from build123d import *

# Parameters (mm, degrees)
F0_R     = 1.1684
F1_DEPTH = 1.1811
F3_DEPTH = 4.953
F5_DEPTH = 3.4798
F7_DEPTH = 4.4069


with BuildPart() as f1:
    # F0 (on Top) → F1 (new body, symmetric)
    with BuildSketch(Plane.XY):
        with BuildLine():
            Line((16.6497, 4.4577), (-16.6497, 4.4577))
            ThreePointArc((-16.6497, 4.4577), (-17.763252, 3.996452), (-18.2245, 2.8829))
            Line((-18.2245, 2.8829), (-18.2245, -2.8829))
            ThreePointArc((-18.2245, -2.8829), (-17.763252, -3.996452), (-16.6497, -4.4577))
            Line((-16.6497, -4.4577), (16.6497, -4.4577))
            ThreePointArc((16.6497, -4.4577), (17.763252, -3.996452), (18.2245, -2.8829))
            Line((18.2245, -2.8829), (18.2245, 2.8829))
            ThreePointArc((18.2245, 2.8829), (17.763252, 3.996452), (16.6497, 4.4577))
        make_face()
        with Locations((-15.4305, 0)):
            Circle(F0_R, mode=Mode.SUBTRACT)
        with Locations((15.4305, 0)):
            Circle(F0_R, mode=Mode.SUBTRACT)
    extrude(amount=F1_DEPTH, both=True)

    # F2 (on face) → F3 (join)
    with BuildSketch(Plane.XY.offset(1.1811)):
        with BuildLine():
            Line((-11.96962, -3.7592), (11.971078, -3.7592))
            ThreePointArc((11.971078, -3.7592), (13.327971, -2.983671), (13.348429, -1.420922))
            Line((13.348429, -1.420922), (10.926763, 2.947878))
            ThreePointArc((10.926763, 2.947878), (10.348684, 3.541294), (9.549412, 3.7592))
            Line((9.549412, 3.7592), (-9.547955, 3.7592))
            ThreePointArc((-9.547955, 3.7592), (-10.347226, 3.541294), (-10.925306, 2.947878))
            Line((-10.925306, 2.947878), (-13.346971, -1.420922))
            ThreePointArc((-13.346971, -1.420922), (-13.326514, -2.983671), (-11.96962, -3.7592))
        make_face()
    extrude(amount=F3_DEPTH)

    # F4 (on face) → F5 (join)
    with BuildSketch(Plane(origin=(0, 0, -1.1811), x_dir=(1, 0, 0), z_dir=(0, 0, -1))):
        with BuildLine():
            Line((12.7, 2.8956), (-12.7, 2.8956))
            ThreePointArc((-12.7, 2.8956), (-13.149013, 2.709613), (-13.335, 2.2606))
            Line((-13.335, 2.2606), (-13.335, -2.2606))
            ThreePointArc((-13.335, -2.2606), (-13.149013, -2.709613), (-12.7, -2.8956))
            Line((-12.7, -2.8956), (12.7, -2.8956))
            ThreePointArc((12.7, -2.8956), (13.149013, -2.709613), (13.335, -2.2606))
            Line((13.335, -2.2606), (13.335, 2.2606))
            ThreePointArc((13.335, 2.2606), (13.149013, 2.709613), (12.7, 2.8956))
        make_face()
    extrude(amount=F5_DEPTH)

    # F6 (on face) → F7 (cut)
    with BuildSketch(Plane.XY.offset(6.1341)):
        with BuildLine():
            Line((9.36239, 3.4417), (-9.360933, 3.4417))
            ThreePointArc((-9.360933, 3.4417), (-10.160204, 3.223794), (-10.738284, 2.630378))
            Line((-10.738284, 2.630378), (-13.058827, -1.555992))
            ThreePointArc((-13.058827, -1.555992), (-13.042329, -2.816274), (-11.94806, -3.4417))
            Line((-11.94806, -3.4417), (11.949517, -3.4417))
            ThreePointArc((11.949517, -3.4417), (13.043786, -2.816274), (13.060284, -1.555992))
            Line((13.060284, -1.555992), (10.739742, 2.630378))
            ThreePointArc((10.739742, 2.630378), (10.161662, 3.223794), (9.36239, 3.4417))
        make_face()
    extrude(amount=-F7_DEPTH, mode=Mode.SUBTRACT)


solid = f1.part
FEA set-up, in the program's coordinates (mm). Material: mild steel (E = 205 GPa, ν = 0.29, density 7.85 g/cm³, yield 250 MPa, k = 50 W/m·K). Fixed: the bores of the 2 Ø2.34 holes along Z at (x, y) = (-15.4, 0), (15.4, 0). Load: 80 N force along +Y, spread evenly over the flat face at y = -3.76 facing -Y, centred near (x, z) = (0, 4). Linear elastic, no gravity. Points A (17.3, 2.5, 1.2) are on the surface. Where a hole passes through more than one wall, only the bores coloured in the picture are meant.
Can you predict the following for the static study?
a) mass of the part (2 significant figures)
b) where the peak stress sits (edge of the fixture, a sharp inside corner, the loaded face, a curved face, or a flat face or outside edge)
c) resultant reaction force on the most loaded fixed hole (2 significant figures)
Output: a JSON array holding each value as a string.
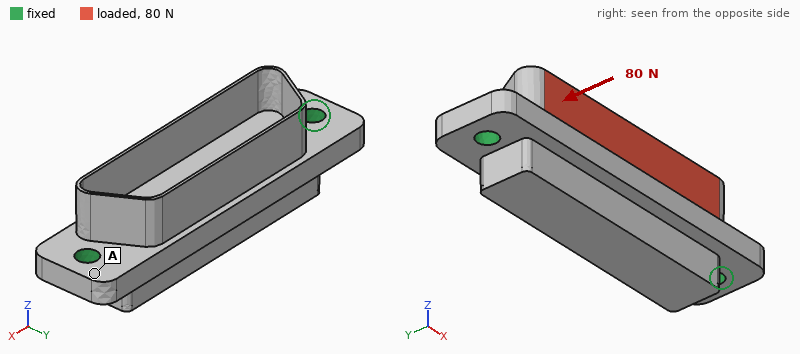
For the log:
["12 g", "the loaded face", "41 N"]
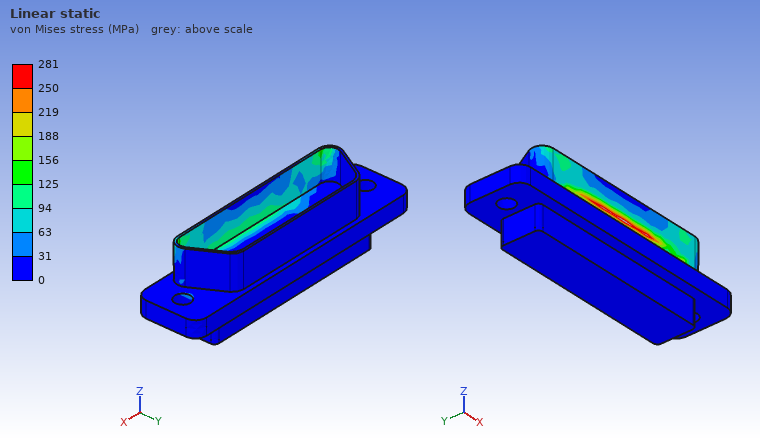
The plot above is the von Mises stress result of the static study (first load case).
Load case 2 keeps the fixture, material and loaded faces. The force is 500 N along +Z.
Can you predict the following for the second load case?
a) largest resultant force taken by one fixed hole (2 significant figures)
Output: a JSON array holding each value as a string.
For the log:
["280 N"]
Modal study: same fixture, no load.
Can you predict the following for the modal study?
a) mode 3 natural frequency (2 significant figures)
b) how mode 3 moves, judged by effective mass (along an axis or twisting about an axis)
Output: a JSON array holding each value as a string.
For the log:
["20 kHz", "along Z"]
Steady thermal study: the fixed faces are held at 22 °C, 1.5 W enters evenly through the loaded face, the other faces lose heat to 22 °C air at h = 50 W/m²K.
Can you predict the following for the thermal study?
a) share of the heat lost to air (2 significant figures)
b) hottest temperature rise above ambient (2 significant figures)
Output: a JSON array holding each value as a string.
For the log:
["15 %", "12 K"]
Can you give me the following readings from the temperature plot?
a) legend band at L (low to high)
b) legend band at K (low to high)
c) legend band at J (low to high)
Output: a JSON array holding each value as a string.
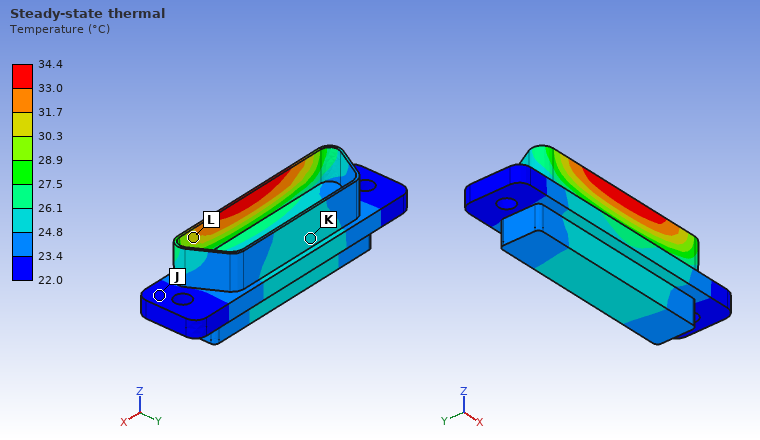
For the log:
["30.3 to 31.7 °C", "24.8 to 26.1 °C", "22.0 to 23.4 °C"]
